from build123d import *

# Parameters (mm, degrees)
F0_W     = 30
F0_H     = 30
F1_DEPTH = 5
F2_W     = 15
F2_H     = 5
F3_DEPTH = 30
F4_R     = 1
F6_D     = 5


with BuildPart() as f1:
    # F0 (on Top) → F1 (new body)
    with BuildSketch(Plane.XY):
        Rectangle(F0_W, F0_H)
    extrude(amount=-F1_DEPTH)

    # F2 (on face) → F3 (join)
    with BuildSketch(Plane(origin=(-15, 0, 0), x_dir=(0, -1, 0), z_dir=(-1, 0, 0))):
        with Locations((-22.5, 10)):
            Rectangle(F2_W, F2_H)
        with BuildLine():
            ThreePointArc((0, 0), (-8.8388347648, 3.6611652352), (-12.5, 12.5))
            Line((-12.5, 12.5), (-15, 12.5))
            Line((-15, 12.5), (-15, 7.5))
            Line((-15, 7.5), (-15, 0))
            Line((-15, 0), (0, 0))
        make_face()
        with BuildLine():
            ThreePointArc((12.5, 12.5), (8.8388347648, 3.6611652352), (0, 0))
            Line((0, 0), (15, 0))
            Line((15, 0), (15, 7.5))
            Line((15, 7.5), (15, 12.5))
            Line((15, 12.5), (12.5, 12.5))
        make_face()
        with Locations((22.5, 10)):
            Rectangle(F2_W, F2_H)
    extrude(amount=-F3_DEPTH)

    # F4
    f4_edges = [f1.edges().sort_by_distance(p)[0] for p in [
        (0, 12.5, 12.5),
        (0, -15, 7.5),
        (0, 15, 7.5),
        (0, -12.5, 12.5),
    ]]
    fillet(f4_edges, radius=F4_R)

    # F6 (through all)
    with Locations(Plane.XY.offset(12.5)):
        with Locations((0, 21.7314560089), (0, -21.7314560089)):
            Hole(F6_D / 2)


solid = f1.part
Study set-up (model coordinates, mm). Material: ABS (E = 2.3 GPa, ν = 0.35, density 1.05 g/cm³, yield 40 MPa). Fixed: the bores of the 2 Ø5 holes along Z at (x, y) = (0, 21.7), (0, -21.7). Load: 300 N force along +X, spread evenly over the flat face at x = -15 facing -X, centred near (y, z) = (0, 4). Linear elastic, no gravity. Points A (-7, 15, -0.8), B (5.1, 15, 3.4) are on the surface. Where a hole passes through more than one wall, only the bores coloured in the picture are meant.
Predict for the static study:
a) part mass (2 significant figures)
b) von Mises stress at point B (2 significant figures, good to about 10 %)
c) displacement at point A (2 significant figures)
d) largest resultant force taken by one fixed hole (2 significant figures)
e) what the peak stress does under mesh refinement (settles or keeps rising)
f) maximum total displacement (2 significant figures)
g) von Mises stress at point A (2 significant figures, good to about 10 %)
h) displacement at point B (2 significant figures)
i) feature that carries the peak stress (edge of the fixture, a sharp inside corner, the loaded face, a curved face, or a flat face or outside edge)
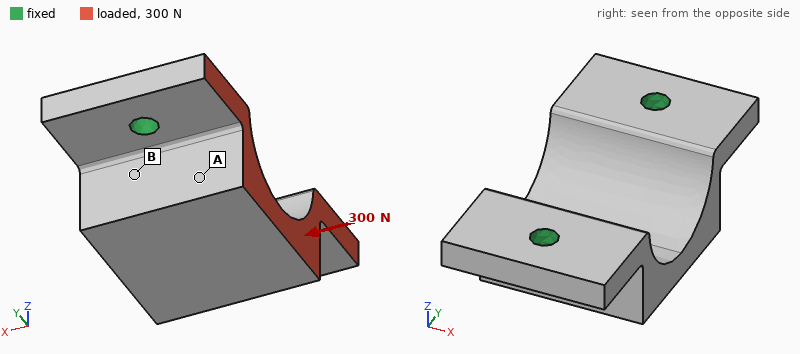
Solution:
13 g
2.4 MPa
0.12 mm
150 N
keeps rising
0.20 mm
1.4 MPa
0.082 mm
edge of the fixture
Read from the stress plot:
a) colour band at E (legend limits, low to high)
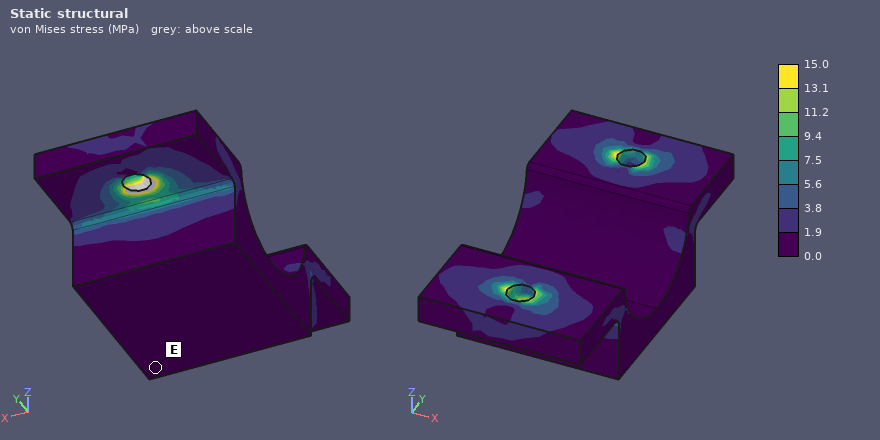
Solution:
0.0 to 1.9 MPa
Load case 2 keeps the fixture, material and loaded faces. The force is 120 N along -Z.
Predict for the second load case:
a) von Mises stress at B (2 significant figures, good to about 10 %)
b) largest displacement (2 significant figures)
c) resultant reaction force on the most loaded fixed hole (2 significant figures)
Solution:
0.99 MPa
0.15 mm
64 N
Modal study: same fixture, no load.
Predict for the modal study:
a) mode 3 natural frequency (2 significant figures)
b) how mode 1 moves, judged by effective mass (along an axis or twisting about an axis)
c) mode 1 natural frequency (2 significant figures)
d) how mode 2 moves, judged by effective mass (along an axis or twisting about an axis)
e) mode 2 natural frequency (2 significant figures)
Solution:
4600 Hz
along X
1800 Hz
along Z
4400 Hz
